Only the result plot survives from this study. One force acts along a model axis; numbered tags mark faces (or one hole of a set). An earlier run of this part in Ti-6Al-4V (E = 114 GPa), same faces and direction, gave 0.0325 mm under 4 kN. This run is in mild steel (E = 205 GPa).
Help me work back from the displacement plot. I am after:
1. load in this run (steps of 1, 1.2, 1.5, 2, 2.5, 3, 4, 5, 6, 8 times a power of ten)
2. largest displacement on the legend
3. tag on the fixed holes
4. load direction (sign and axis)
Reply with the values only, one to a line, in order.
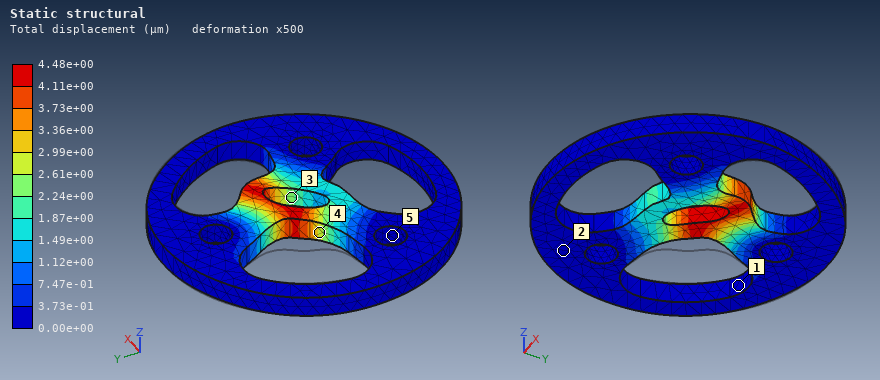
1 kN
4.48e+00 µm
5
+X
